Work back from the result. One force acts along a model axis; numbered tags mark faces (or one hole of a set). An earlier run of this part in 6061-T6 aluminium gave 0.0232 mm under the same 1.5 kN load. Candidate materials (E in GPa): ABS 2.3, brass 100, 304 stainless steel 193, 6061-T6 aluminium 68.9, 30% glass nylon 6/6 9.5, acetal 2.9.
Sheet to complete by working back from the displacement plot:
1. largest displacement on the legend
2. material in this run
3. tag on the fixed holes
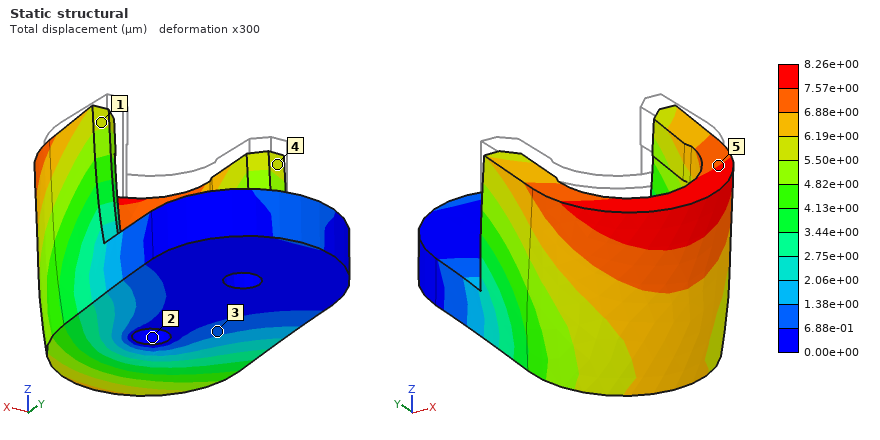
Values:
8.26e+00 µm
304 stainless steel
2
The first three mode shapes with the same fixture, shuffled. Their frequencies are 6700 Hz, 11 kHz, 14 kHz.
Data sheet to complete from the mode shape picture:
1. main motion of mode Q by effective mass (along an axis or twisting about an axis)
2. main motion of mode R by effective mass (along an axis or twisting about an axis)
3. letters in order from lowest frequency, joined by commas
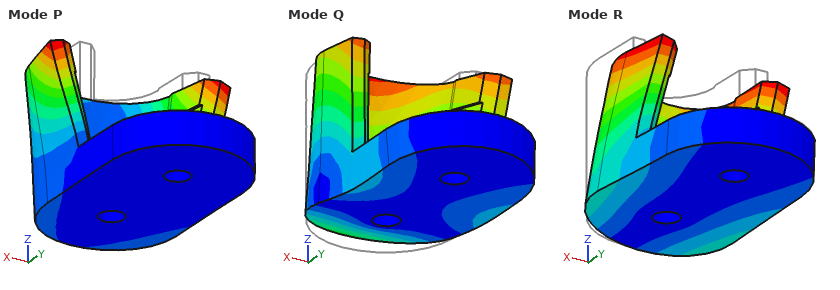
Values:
along Y
along X
R, Q, P
